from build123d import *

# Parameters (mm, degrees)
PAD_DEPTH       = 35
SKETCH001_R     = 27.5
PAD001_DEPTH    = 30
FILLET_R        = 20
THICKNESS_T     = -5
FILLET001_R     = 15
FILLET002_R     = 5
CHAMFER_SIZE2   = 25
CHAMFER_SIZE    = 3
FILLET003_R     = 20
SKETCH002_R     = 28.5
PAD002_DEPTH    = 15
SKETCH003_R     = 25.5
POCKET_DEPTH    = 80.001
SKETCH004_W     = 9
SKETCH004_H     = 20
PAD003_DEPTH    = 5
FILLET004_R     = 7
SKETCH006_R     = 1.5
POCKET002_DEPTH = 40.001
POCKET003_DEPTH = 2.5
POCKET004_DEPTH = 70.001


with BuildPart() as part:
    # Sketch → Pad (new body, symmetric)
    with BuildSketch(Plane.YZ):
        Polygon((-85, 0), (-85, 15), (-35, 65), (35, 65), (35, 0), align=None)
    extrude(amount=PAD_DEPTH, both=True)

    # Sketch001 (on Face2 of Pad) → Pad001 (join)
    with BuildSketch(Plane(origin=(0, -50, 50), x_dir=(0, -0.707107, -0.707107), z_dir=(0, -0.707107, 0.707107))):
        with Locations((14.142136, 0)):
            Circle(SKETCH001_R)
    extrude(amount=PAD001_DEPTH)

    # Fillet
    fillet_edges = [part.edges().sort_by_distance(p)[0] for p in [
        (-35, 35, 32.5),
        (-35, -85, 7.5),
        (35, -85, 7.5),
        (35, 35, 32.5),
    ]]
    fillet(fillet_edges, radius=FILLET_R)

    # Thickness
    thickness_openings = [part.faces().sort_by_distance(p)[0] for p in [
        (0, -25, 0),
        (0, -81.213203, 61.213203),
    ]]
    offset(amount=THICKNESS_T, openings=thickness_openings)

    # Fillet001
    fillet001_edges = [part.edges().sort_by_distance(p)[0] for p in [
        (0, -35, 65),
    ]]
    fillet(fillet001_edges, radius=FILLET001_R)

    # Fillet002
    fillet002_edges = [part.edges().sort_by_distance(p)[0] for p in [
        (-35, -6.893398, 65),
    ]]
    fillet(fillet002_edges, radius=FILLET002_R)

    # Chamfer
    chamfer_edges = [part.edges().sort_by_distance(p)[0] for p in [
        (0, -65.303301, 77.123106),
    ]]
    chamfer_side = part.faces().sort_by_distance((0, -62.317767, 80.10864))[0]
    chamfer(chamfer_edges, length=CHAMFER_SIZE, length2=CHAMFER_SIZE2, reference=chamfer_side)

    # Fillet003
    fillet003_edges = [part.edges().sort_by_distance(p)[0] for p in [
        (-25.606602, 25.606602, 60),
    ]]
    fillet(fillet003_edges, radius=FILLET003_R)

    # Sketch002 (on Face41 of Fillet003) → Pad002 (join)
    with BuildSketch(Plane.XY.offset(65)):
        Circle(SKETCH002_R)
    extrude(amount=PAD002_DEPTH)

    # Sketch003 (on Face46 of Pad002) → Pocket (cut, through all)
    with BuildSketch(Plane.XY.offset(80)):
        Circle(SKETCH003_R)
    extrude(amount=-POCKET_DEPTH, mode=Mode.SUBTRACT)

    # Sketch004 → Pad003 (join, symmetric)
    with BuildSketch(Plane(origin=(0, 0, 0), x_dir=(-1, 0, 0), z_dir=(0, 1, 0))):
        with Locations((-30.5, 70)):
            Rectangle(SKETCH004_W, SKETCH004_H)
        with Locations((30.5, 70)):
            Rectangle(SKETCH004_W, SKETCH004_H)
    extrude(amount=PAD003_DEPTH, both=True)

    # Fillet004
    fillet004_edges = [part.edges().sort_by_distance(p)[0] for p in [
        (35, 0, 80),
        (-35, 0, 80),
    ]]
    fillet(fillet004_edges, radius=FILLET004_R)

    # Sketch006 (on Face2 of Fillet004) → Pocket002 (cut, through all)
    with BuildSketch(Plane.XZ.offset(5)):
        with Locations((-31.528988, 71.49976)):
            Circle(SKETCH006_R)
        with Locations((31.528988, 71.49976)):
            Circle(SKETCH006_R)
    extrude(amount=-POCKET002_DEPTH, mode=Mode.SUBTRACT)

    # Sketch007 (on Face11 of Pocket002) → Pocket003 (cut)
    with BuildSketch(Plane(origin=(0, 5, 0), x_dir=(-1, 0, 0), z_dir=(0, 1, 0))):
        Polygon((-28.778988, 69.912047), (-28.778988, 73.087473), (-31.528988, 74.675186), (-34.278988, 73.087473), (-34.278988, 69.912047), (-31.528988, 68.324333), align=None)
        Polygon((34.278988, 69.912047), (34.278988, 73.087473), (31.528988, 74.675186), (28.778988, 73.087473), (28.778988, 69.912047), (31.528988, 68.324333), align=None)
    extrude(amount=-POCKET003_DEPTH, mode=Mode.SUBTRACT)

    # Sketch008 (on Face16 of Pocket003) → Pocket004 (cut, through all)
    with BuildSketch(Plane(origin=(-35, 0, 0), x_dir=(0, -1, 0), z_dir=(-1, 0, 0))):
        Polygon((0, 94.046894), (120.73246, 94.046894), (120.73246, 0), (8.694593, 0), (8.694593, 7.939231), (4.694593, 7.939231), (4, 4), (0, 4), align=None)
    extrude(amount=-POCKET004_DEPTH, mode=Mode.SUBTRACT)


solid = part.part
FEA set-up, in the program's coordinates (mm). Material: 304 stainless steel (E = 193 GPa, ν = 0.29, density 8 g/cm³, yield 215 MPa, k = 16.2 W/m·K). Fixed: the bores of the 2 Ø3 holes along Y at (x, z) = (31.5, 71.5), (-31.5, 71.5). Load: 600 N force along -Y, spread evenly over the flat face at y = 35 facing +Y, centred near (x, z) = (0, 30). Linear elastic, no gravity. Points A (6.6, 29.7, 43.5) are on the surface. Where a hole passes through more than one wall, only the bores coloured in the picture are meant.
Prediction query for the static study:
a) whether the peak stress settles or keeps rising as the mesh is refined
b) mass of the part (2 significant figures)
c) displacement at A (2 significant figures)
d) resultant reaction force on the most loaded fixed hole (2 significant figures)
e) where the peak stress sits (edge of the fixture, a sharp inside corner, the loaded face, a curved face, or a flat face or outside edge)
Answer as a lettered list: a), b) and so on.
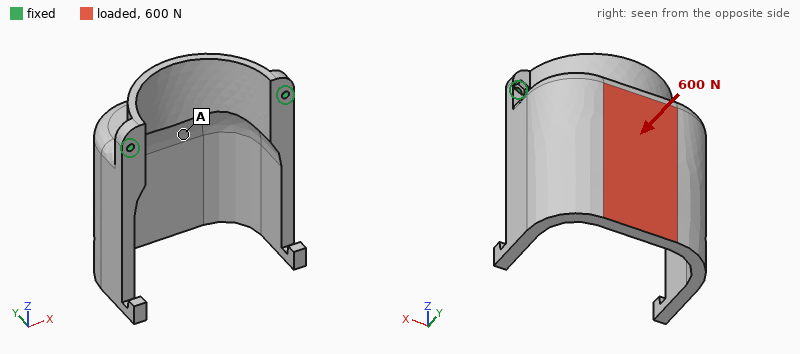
a) keeps rising
b) 410 g
c) 0.20 mm
d) 300 N
e) edge of the fixture
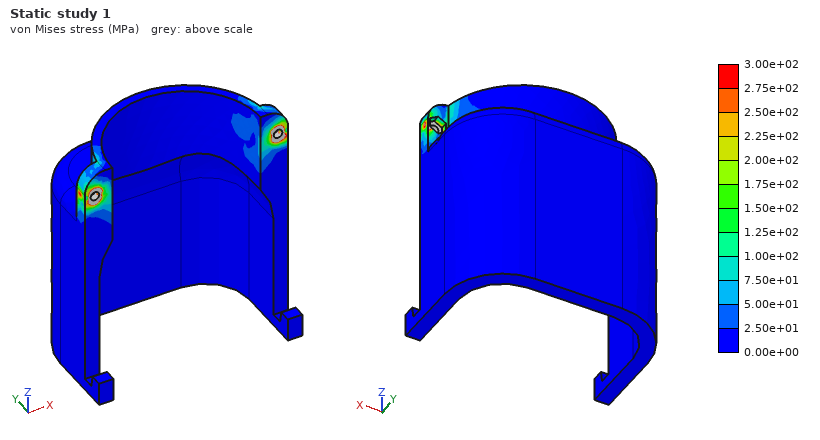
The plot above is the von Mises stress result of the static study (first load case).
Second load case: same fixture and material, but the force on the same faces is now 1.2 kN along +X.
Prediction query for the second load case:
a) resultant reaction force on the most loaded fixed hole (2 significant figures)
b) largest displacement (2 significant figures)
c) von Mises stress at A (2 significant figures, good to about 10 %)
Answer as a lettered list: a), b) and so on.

a) 1.1 kN
b) 59 µm
c) 17 MPa
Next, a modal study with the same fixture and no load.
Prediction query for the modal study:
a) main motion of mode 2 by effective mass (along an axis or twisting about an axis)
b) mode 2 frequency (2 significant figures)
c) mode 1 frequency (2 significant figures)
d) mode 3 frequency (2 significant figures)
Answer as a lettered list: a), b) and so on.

a) along X
b) 1200 Hz
c) 400 Hz
d) 2800 Hz
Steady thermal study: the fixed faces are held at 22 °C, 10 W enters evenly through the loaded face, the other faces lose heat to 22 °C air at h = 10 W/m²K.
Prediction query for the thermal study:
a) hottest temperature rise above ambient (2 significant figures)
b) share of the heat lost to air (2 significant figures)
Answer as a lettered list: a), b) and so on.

a) 55 K
b) 62 %
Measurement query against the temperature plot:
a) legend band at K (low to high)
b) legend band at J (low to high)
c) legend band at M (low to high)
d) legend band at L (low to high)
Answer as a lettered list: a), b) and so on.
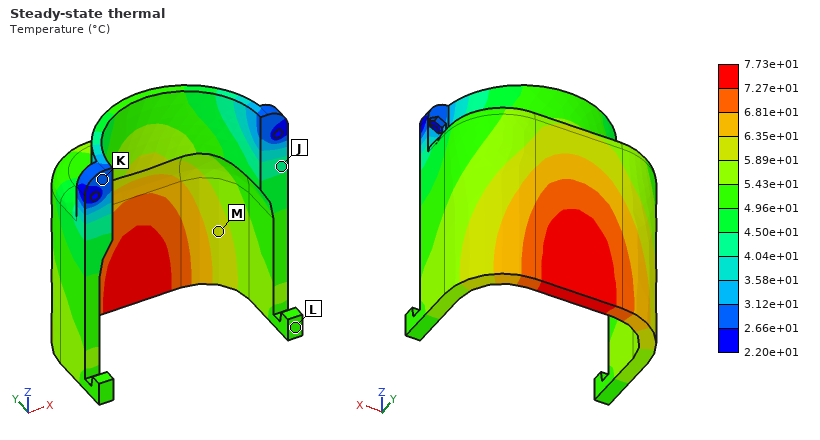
a) 2.66e+01 to 3.12e+01 °C
b) 4.04e+01 to 4.50e+01 °C
c) 5.89e+01 to 6.35e+01 °C
d) 4.96e+01 to 5.43e+01 °C
